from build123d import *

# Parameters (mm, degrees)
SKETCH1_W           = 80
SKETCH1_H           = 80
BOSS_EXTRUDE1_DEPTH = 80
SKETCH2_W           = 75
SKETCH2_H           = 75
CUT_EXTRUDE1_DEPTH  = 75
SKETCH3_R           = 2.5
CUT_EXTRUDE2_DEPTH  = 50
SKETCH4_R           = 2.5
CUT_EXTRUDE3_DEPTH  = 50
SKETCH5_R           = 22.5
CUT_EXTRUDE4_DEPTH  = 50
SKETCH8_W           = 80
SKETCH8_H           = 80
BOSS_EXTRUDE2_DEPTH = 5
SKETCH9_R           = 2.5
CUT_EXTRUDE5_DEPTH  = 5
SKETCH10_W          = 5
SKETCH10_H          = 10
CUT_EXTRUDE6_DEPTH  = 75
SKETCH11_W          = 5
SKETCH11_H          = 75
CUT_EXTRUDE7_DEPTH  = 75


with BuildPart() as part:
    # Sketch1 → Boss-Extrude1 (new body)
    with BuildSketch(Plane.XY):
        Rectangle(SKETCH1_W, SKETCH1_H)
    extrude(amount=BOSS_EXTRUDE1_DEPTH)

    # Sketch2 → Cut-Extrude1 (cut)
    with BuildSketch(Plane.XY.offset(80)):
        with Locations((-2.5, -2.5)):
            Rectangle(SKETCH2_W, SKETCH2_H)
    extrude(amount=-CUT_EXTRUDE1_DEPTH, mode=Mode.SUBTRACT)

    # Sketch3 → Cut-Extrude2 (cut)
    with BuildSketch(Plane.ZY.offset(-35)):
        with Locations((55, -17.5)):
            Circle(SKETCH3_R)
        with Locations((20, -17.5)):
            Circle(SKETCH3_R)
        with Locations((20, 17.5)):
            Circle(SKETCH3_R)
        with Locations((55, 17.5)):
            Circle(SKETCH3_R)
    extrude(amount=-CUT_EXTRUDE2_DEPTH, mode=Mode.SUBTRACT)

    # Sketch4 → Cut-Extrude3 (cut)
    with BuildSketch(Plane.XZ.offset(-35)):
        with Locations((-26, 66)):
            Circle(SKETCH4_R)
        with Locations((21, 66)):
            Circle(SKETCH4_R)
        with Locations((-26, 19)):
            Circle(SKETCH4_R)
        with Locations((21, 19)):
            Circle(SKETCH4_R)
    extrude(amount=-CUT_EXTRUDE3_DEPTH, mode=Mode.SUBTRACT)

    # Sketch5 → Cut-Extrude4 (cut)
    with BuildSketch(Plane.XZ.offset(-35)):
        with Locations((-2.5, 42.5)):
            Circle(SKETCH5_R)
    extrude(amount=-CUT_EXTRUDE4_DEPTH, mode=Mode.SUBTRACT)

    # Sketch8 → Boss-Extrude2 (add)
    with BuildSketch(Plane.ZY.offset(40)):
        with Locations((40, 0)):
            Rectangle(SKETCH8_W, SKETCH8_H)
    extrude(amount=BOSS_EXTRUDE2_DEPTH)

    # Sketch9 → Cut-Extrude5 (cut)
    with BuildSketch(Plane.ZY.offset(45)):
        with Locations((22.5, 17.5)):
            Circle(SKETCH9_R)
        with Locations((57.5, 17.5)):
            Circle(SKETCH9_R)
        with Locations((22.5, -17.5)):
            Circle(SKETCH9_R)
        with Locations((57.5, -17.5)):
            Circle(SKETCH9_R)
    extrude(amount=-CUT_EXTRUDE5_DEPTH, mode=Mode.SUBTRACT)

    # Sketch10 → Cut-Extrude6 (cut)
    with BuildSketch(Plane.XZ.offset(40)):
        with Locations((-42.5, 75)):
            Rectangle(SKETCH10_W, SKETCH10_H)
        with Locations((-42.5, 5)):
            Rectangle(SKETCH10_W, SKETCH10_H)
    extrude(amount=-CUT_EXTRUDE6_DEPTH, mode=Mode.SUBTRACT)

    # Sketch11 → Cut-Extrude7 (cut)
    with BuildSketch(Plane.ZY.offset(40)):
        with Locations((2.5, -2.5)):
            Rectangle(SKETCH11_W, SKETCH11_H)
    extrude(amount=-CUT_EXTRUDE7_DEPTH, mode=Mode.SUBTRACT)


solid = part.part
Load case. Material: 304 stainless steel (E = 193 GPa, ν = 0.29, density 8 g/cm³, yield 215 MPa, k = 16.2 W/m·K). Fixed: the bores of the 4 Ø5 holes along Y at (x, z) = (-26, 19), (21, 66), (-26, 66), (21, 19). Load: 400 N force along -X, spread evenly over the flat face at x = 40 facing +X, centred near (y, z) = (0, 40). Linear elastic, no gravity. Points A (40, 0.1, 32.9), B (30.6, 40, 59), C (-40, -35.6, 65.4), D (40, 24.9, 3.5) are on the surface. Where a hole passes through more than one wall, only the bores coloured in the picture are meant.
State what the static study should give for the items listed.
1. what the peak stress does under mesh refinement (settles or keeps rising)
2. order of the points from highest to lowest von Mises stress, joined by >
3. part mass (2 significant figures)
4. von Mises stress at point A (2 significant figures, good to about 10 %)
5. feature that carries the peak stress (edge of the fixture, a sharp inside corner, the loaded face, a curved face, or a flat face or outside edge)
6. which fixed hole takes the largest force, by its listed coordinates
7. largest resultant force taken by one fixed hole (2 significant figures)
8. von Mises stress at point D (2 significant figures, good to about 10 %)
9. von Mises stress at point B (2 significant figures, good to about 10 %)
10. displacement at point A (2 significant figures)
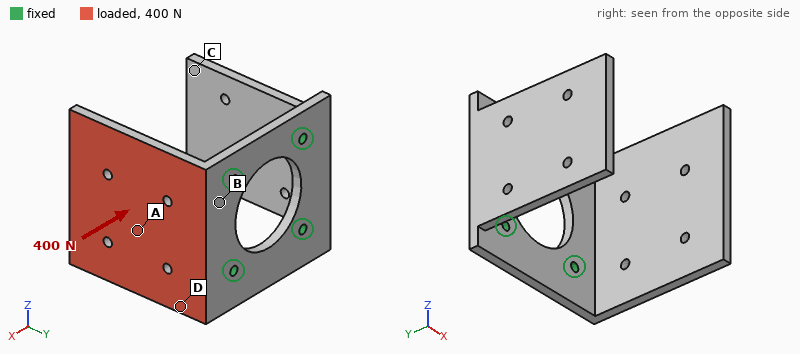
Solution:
keeps rising
B > D > A > C
620 g
11 MPa
edge of the fixture
(21, 19)
230 N
33 MPa
42 MPa
0.11 mm
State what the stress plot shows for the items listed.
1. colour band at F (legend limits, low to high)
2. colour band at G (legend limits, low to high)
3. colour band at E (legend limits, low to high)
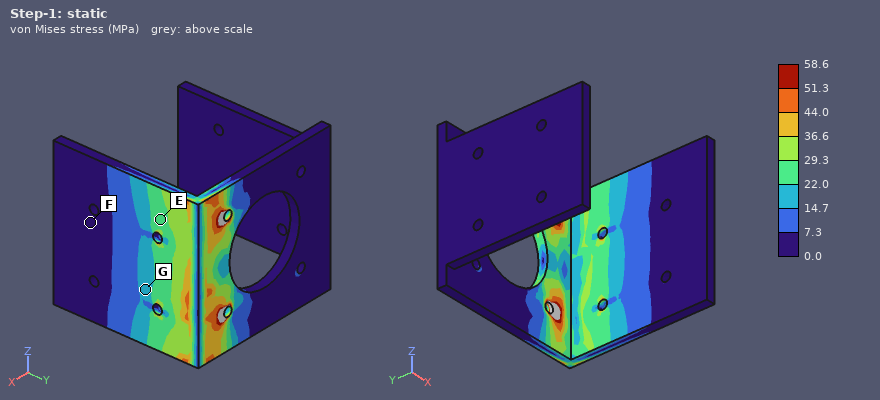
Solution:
0.0 to 7.3 MPa
14.7 to 22.0 MPa
22.0 to 29.3 MPa
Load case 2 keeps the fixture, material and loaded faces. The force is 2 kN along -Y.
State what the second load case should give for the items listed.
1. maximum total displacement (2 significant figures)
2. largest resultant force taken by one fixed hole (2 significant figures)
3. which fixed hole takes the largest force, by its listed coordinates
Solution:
0.27 mm
1.2 kN
(21, 19)
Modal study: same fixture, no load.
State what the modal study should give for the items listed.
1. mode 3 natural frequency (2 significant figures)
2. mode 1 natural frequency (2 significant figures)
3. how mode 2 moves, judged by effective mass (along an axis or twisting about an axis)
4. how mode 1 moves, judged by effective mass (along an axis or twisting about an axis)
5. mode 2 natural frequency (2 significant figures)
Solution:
1300 Hz
480 Hz
along X
along X
510 Hz
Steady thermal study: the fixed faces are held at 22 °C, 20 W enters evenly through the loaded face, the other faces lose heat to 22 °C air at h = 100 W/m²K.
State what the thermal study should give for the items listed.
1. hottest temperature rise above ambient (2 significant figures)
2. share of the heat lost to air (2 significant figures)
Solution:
25 K
87 %
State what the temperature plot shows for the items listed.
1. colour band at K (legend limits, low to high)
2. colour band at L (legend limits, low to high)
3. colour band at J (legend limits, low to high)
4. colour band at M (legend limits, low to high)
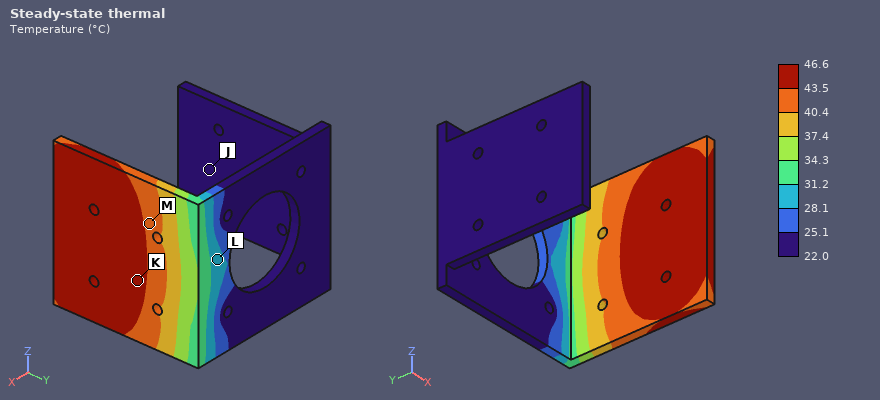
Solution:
43.5 to 46.6 °C
28.1 to 31.2 °C
22.0 to 25.1 °C
40.4 to 43.5 °C
